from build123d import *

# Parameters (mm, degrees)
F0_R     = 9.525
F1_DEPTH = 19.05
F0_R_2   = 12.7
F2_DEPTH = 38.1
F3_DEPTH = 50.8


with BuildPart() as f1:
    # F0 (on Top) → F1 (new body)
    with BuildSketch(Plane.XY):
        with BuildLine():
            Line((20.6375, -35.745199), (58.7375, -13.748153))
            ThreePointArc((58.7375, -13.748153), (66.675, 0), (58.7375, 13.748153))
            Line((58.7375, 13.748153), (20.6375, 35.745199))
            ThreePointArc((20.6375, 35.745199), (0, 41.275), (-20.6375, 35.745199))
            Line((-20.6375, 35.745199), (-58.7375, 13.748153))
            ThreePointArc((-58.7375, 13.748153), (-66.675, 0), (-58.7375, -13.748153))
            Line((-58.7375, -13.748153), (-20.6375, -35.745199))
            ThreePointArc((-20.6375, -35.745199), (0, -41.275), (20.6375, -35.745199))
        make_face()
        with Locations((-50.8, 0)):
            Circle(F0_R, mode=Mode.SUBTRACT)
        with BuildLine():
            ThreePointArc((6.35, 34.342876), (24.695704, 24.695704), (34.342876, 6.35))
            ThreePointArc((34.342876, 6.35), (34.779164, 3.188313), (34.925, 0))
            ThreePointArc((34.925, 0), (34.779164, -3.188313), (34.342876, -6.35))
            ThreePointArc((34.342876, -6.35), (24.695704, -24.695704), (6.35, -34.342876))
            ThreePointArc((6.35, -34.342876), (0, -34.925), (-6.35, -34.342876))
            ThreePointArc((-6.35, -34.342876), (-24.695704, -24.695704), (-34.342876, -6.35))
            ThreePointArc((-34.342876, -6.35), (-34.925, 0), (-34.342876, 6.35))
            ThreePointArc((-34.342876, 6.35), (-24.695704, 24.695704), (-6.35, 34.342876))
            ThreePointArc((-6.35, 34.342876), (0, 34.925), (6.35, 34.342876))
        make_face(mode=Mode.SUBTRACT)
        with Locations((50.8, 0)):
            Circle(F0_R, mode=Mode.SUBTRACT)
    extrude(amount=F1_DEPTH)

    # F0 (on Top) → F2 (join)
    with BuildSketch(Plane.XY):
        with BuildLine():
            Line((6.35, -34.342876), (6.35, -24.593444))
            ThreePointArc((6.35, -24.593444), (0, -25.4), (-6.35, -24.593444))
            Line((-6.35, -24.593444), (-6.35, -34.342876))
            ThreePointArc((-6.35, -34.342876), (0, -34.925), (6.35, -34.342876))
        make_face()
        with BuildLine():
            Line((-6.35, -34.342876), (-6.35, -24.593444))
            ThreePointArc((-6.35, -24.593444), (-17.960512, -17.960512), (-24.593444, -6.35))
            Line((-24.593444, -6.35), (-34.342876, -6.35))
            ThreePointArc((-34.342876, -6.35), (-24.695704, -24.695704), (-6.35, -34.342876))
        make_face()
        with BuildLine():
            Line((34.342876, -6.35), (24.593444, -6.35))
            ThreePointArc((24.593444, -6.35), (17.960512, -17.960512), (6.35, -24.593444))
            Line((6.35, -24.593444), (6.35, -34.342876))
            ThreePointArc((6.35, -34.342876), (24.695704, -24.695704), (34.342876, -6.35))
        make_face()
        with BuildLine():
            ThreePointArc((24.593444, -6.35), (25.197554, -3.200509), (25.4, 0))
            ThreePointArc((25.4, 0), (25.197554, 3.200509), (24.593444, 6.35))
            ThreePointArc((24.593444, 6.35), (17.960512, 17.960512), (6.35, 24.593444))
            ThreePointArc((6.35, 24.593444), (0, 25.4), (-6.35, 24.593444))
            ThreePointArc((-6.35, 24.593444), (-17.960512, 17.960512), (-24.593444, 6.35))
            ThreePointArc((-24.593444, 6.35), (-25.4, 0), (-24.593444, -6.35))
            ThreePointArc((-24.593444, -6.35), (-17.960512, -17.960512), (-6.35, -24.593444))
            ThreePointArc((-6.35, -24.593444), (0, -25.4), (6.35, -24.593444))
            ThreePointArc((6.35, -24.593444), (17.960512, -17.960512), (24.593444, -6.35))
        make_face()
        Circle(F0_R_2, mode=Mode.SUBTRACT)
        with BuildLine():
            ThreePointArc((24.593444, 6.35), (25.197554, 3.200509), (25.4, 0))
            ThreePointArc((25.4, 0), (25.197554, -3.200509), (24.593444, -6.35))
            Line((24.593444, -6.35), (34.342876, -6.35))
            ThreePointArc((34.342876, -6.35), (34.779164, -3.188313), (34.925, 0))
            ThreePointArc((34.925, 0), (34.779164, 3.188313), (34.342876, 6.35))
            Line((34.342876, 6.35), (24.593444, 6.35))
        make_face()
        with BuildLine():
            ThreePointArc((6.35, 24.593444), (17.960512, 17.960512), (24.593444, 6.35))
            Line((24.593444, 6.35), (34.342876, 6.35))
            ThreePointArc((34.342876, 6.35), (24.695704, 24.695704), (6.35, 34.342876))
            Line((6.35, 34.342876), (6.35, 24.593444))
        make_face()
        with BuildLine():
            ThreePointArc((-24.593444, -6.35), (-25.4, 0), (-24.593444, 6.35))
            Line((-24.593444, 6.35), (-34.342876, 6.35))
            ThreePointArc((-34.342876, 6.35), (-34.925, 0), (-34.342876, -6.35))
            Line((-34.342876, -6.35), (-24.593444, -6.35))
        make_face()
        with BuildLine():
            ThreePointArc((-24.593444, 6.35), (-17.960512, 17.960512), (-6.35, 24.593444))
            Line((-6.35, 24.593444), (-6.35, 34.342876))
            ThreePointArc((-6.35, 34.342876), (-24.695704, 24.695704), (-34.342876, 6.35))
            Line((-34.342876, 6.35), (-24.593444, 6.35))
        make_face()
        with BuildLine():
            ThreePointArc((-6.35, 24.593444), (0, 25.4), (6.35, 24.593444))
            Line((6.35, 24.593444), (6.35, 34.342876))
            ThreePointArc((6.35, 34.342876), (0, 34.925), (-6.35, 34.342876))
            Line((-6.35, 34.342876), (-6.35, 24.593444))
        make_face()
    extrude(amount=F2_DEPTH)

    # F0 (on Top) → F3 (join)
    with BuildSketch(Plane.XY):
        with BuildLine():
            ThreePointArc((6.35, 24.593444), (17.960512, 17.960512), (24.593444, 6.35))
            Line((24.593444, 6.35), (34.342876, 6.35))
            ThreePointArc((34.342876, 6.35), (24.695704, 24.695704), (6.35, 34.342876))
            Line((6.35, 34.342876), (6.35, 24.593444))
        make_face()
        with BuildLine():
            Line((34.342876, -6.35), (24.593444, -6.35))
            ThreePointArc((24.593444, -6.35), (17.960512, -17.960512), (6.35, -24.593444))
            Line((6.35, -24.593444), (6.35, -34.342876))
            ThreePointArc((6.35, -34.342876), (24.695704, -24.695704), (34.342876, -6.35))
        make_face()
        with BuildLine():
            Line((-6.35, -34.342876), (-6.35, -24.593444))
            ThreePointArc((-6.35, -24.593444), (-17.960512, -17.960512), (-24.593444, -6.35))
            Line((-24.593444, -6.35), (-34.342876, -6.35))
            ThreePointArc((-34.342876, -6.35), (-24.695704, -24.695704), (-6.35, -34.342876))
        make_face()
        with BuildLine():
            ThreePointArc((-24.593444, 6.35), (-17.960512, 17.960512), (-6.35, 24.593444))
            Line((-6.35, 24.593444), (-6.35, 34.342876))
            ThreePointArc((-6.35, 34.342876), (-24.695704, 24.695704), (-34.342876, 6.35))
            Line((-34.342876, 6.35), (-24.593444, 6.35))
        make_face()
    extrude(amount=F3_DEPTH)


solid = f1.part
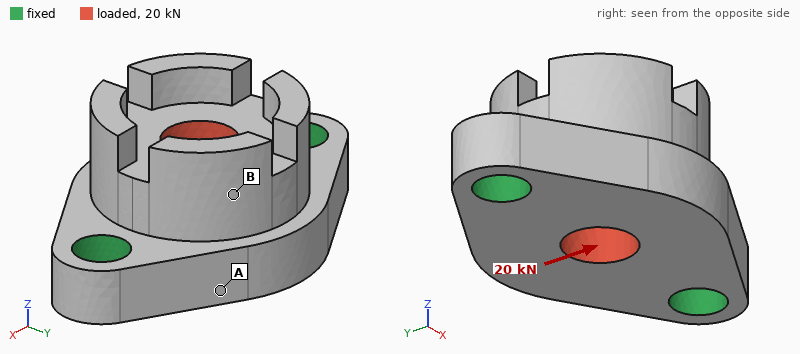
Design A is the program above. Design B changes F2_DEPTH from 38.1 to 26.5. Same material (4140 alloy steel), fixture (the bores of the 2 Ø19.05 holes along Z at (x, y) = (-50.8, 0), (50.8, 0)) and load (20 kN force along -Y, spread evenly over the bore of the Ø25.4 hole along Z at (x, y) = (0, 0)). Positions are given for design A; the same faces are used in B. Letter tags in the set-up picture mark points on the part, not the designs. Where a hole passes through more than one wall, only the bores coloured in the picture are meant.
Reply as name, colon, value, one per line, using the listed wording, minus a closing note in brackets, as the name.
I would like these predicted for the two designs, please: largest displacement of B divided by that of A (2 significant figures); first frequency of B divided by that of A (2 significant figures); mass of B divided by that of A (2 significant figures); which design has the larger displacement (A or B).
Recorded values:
largest displacement of B divided by that of A: 0.55
first frequency of B divided by that of A: 1.0
mass of B divided by that of A: 0.88
which design has the larger displacement: A
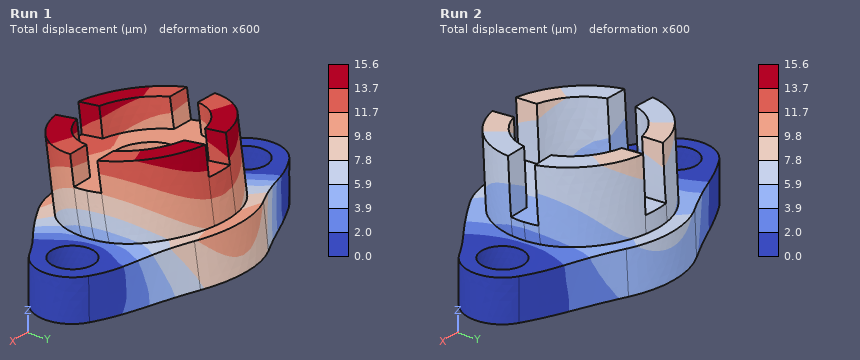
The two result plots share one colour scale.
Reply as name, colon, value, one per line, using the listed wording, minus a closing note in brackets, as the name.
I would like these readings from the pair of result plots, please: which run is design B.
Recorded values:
which run is design B: Run 2
